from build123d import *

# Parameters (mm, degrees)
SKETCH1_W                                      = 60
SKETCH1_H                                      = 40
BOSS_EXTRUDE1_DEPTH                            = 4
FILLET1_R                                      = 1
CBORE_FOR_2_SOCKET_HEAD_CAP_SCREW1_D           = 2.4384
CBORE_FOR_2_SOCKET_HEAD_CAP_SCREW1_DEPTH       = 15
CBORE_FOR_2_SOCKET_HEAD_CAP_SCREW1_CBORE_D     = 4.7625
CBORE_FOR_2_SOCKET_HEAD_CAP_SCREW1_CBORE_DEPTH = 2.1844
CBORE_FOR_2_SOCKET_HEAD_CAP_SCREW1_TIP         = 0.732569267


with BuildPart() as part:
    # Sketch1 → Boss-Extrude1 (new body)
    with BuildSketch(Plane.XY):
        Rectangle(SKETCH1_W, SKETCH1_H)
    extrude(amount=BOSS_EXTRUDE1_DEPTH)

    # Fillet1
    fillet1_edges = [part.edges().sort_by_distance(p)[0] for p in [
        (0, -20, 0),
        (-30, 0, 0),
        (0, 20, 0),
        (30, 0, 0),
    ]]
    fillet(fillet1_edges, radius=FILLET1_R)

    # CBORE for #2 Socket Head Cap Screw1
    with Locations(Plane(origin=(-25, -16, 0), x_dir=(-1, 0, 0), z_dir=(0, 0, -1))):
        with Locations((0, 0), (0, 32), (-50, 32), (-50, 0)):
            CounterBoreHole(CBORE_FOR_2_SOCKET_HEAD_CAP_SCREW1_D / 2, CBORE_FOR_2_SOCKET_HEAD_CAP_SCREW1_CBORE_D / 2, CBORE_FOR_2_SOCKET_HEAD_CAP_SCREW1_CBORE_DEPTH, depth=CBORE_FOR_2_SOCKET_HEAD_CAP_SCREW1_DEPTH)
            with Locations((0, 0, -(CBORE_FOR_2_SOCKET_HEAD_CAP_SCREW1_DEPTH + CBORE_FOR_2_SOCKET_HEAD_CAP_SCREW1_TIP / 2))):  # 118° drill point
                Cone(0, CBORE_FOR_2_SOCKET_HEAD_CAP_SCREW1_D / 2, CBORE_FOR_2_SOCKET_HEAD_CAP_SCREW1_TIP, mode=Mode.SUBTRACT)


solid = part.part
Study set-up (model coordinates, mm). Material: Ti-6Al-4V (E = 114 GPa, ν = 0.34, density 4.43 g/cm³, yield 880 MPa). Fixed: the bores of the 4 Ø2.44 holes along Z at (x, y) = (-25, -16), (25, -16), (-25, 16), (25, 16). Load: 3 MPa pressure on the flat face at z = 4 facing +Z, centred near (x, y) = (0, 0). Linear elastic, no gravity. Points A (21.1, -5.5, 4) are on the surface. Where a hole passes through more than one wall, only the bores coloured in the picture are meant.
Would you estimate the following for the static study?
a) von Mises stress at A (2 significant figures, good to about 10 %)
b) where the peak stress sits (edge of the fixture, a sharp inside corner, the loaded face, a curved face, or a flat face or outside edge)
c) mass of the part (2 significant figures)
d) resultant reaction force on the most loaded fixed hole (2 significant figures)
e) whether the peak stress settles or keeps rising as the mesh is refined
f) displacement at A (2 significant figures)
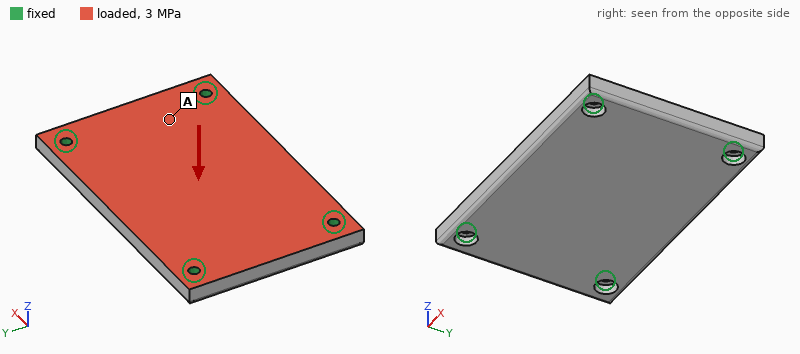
61 MPa
edge of the fixture
41 g
2.8 kN
keeps rising
0.068 mm
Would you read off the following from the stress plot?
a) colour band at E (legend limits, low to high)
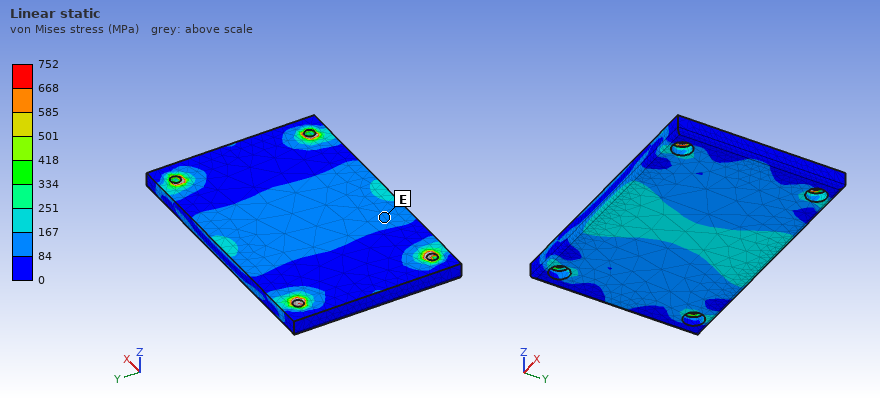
84 to 167 MPa
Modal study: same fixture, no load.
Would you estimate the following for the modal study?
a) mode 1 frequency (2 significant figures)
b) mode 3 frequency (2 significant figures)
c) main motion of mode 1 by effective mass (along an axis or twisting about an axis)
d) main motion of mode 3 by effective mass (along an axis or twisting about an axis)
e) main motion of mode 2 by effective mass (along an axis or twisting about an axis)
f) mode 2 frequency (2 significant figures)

5400 Hz
13 kHz
along Z
twisting about Y
twisting about X
8700 Hz
